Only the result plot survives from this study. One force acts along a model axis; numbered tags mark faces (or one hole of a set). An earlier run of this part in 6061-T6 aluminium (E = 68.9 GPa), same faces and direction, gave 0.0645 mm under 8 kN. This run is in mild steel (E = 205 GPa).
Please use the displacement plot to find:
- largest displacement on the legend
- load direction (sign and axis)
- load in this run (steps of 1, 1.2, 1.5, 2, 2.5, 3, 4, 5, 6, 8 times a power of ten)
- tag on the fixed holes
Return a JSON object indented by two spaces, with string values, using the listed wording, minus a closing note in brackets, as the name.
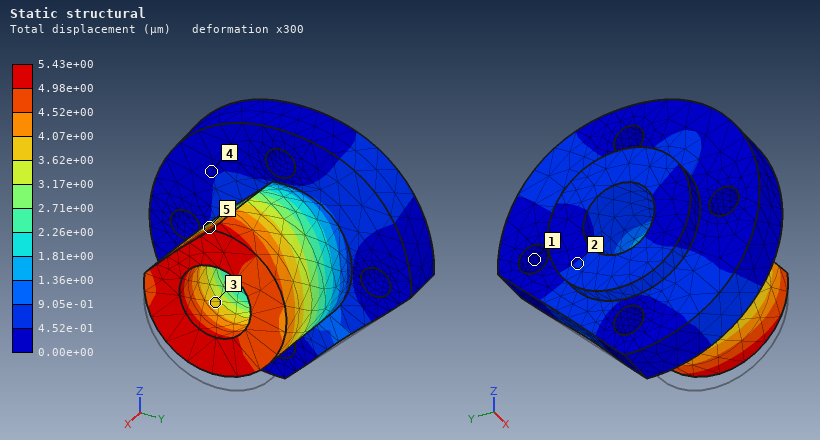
{
  "largest displacement on the legend": "5.43e+00 µm",
  "load direction": "+Z",
  "load in this run": "2 kN",
  "tag on the fixed holes": "1"
}
